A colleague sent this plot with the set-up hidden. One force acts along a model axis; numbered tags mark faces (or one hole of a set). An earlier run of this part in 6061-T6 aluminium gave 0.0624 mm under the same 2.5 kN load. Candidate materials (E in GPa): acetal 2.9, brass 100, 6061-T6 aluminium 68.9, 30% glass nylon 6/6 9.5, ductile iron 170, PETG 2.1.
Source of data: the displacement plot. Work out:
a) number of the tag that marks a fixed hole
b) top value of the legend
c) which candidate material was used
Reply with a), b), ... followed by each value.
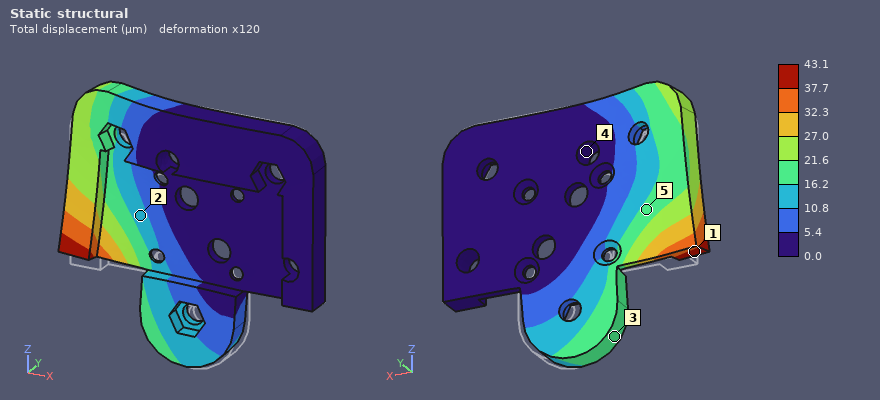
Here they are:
a) 4
b) 43.1 µm
c) brass
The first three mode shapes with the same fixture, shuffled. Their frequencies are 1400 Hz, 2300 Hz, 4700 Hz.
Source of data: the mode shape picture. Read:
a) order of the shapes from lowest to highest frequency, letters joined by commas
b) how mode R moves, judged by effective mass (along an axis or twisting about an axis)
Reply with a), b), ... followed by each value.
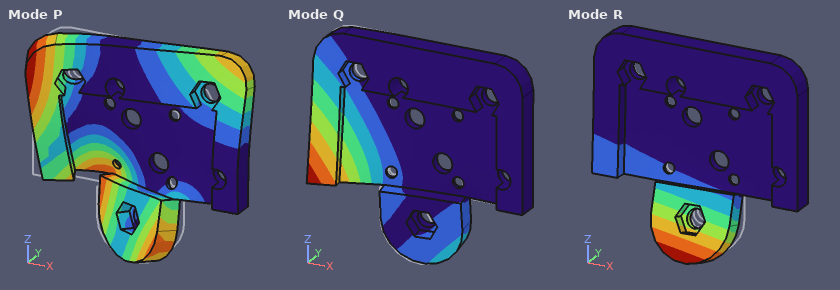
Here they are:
a) R, Q, P
b) along Y
